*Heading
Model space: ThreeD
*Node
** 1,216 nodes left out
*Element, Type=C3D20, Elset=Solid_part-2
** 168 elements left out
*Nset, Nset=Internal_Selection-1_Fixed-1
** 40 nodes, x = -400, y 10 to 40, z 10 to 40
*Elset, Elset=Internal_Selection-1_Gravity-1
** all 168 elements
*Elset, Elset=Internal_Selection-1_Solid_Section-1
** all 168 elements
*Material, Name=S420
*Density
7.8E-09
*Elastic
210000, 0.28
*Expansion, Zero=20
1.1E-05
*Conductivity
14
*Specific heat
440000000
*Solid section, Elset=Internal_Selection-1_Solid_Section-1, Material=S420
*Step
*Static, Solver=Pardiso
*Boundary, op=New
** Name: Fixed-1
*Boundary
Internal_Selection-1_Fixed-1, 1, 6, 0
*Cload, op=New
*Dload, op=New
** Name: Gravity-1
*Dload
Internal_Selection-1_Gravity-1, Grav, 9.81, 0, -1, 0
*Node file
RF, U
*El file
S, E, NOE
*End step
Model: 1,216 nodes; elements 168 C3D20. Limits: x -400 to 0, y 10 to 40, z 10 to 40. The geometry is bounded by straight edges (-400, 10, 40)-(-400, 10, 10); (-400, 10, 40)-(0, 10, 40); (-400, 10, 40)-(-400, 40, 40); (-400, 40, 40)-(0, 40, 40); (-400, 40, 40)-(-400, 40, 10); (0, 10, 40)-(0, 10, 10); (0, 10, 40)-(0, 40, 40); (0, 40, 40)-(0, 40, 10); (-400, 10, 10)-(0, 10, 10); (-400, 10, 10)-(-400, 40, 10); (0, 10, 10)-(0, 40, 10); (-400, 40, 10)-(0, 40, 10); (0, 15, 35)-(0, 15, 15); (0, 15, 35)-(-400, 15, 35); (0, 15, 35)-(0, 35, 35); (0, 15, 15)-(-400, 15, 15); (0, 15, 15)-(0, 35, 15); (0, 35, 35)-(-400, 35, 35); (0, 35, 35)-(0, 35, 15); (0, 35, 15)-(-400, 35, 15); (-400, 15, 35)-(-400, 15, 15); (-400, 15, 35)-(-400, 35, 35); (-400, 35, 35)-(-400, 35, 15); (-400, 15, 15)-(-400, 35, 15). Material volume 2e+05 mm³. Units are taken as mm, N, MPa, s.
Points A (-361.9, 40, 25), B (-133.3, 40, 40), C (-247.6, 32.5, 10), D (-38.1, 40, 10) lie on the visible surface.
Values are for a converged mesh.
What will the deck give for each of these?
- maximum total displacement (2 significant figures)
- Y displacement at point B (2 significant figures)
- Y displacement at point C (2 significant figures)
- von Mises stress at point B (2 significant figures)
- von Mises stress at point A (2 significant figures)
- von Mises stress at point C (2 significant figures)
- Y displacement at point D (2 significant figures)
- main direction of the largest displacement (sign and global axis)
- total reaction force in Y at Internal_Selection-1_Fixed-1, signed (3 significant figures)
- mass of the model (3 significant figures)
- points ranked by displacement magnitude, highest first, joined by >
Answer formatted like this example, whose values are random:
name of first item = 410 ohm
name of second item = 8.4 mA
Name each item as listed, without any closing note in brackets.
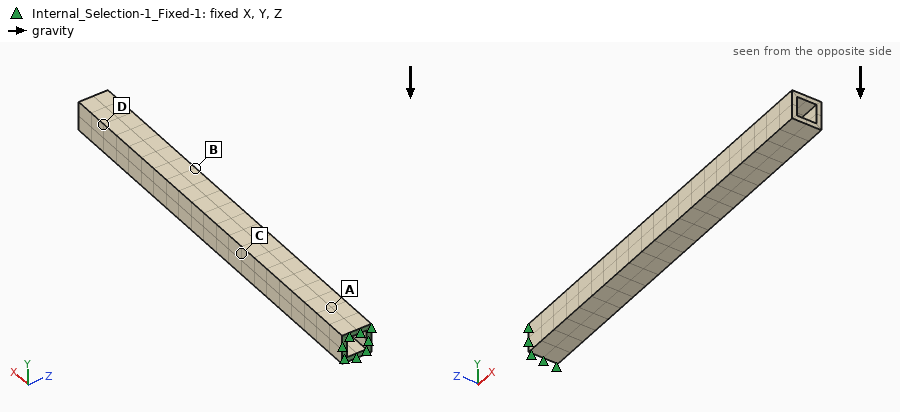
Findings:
maximum total displacement = 1.1e-05 mm
Y displacement at point B = -6.1e-06 mm
Y displacement at point C = -2.5e-06 mm
von Mises stress at point B = 9.3e-05 MPa
von Mises stress at point A = 7.0e-04 MPa
von Mises stress at point C = 1.8e-04 MPa
Y displacement at point D = -9.5e-06 mm
main direction of the largest displacement = -Y
total reaction force in Y at Internal_Selection-1_Fixed-1, signed = 0.0153 N
mass of the model = 1.56 kg
points ranked by displacement magnitude, highest first, joined by > = D > B > C > A
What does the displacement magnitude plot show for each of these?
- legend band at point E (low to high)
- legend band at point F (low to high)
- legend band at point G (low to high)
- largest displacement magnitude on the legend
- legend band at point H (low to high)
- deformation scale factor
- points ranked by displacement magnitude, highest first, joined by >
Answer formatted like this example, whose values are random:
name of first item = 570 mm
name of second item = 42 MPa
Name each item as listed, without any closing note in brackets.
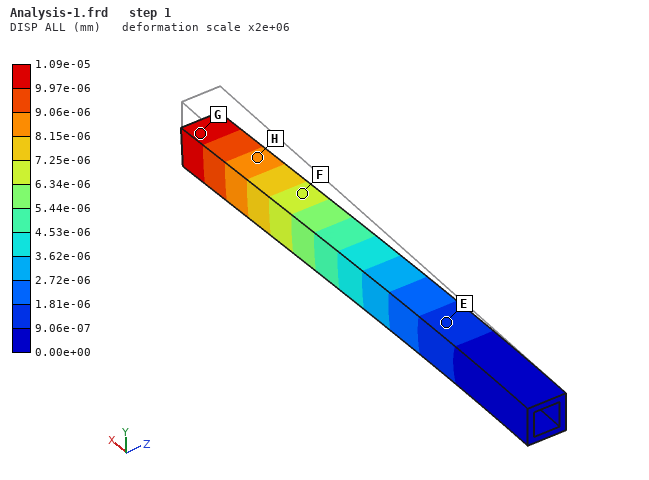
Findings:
legend band at point E = 9.06e-07 to 1.81e-06 mm
legend band at point F = 6.34e-06 to 7.25e-06 mm
legend band at point G = 9.97e-06 to 1.09e-05 mm
largest displacement magnitude on the legend = 1.09e-05 mm
legend band at point H = 8.15e-06 to 9.06e-06 mm
deformation scale factor = 2e+06
points ranked by displacement magnitude, highest first, joined by > = G > H > F > E
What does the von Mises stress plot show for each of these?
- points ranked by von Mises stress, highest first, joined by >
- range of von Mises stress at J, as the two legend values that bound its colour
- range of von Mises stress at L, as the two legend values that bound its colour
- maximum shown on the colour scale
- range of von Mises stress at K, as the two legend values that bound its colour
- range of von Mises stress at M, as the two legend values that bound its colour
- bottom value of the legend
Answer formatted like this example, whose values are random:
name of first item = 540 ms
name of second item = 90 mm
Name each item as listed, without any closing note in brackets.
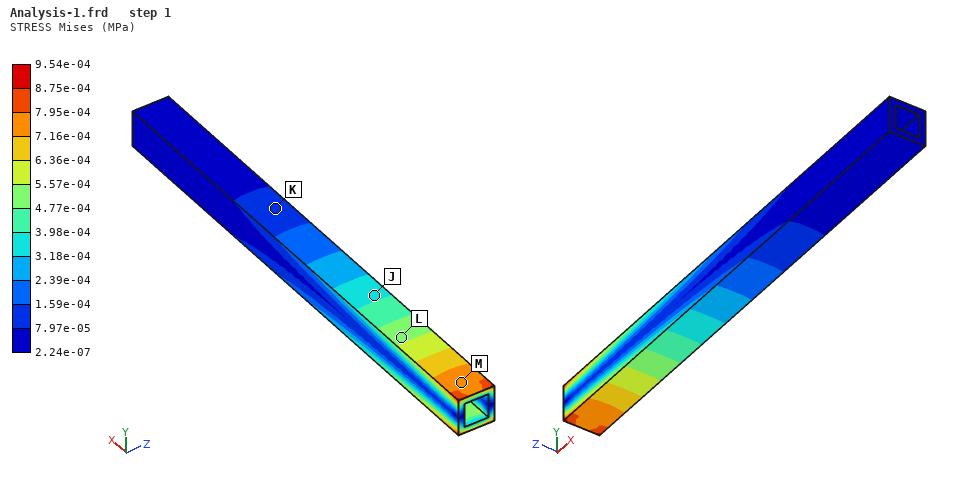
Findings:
points ranked by von Mises stress, highest first, joined by > = M > L > J > K
range of von Mises stress at J, as the two legend values that bound its colour = 3.18e-04 to 3.98e-04 MPa
range of von Mises stress at L, as the two legend values that bound its colour = 4.77e-04 to 5.57e-04 MPa
maximum shown on the colour scale = 9.54e-04 MPa
range of von Mises stress at K, as the two legend values that bound its colour = 7.97e-05 to 1.59e-04 MPa
range of von Mises stress at M, as the two legend values that bound its colour = 7.16e-04 to 7.95e-04 MPa
bottom value of the legend = 2.24e-07 MPa
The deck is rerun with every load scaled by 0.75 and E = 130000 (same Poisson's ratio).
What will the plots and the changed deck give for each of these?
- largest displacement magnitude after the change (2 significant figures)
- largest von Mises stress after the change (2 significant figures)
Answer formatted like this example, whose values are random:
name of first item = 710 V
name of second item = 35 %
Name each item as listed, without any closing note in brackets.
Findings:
largest displacement magnitude after the change = 1.3e-05 mm
largest von Mises stress after the change = 7.2e-04 MPa
